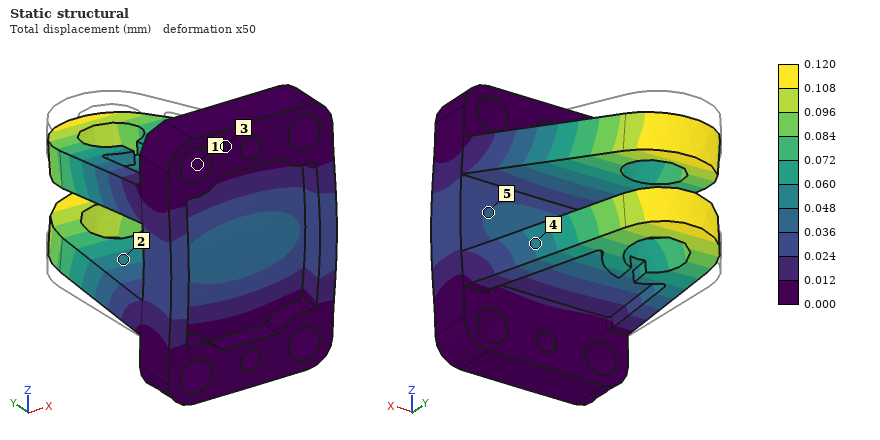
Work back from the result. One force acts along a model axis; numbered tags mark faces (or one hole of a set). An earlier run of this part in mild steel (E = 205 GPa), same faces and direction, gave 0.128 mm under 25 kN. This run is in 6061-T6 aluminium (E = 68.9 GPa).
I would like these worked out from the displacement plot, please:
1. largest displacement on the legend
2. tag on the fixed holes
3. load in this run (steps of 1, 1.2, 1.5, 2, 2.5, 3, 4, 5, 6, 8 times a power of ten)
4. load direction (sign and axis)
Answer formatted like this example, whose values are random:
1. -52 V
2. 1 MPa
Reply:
1. 0.120 mm
2. 1
3. 8 kN
4. -Y
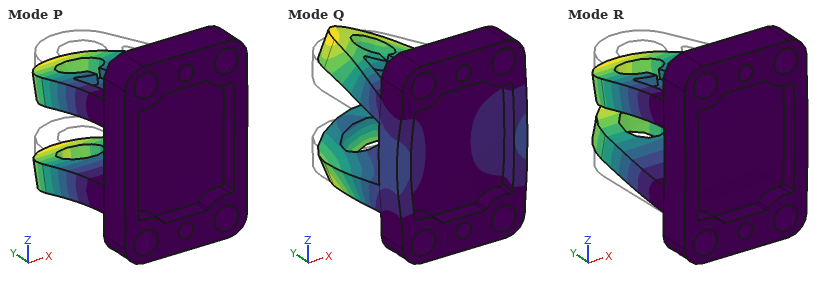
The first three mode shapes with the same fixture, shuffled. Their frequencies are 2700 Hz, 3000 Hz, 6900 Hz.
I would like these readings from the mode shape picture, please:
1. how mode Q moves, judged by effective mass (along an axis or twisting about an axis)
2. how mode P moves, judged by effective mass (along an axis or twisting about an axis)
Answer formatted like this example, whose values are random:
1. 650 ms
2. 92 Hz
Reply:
1. along X
2. along Z
